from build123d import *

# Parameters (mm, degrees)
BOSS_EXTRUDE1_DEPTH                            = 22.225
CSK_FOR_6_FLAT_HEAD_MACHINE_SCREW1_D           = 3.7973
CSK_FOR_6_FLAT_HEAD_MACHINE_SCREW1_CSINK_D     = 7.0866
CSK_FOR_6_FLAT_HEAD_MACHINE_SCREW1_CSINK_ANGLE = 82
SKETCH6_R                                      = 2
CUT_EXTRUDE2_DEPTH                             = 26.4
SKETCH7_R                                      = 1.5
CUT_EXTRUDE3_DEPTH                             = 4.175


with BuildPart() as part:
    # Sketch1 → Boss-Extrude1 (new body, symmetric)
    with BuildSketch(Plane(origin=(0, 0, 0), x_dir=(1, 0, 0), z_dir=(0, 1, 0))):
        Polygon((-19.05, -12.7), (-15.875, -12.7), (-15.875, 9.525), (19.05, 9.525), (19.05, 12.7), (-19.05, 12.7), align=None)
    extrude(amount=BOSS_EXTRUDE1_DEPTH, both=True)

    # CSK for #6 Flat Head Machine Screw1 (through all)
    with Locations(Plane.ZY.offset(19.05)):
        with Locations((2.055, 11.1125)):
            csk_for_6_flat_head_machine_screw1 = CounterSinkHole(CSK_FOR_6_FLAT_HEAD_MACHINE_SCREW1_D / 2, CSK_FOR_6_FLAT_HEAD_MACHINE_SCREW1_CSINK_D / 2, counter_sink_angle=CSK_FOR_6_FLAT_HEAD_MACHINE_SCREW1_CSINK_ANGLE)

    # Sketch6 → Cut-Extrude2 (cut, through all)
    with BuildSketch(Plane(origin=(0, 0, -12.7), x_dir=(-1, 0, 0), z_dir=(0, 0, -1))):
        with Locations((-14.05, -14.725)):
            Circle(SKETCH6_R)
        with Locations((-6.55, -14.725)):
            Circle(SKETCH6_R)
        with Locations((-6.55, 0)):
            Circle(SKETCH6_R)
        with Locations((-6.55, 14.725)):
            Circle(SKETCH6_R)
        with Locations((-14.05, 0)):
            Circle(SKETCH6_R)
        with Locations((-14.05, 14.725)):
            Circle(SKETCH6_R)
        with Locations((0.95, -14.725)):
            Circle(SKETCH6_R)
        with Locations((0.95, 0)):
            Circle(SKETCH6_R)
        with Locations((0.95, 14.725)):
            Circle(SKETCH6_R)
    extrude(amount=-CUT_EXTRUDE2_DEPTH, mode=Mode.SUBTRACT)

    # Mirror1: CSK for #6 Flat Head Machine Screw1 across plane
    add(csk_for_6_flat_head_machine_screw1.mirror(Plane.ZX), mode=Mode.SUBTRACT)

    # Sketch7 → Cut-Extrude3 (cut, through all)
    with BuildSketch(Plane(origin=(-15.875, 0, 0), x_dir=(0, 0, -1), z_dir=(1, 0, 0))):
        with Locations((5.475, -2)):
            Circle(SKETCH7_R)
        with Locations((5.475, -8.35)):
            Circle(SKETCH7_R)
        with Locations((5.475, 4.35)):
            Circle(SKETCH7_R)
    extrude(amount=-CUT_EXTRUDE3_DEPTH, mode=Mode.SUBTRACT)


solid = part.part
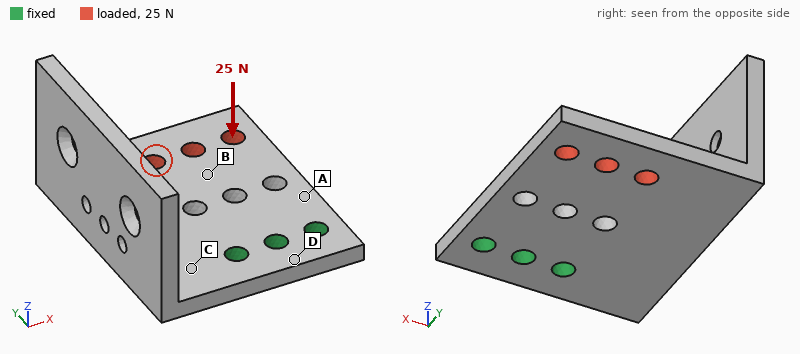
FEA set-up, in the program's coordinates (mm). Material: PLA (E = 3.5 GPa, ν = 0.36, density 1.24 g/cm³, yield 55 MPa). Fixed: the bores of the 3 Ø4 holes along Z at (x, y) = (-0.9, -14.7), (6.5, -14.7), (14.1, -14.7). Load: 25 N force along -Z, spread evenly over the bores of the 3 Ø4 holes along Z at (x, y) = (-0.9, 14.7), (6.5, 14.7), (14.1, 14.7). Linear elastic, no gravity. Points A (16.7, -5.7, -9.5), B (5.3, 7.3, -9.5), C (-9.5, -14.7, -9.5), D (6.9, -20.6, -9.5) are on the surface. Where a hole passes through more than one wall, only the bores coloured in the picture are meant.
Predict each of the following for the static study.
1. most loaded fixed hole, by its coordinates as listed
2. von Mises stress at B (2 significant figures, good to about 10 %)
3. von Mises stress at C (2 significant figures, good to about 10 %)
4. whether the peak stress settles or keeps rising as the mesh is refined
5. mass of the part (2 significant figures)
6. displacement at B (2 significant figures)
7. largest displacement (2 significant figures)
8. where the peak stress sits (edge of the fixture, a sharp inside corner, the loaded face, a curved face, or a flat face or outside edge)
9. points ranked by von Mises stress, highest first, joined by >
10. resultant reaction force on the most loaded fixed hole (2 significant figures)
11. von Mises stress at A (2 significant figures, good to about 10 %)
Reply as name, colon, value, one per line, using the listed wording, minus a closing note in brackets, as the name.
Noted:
most loaded fixed hole, by its coordinates as listed: (6.5, -14.7)
von Mises stress at B: 2.8 MPa
von Mises stress at C: 5.8 MPa
whether the peak stress settles or keeps rising as the mesh is refined: keeps rising
mass of the part: 9.9 g
displacement at B: 0.32 mm
largest displacement: 0.76 mm
where the peak stress sits: edge of the fixture
points ranked by von Mises stress, highest first, joined by >: A > C > B > D
resultant reaction force on the most loaded fixed hole: 13 N
von Mises stress at A: 8.1 MPa
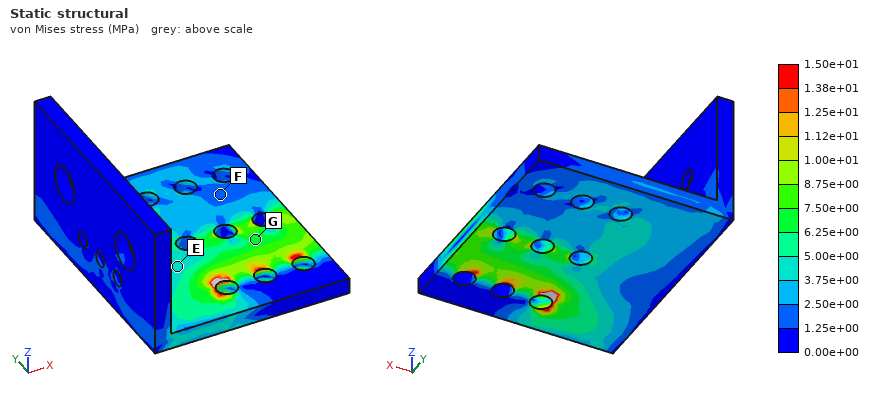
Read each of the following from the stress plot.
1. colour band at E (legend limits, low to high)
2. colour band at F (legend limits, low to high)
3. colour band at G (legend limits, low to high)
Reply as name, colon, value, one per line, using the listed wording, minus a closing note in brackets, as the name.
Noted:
colour band at E: 3.75e+00 to 5.00e+00 MPa
colour band at F: 1.25e+00 to 2.50e+00 MPa
colour band at G: 6.25e+00 to 7.50e+00 MPa
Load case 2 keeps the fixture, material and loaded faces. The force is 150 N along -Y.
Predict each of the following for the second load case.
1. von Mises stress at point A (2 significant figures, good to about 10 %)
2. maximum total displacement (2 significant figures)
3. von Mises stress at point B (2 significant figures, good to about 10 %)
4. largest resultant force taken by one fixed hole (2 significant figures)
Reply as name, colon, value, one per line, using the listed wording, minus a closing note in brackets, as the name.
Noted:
von Mises stress at point A: 2.1 MPa
maximum total displacement: 22 µm
von Mises stress at point B: 2.0 MPa
largest resultant force taken by one fixed hole: 58 N
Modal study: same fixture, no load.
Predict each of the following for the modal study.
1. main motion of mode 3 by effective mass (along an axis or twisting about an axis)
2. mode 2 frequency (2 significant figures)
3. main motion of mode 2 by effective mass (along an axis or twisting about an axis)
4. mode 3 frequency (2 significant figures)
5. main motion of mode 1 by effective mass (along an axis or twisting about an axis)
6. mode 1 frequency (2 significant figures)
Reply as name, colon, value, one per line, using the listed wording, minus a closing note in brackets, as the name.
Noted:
main motion of mode 3 by effective mass: along Z
mode 2 frequency: 680 Hz
main motion of mode 2 by effective mass: along X
mode 3 frequency: 1300 Hz
main motion of mode 1 by effective mass: along Z
mode 1 frequency: 440 Hz
